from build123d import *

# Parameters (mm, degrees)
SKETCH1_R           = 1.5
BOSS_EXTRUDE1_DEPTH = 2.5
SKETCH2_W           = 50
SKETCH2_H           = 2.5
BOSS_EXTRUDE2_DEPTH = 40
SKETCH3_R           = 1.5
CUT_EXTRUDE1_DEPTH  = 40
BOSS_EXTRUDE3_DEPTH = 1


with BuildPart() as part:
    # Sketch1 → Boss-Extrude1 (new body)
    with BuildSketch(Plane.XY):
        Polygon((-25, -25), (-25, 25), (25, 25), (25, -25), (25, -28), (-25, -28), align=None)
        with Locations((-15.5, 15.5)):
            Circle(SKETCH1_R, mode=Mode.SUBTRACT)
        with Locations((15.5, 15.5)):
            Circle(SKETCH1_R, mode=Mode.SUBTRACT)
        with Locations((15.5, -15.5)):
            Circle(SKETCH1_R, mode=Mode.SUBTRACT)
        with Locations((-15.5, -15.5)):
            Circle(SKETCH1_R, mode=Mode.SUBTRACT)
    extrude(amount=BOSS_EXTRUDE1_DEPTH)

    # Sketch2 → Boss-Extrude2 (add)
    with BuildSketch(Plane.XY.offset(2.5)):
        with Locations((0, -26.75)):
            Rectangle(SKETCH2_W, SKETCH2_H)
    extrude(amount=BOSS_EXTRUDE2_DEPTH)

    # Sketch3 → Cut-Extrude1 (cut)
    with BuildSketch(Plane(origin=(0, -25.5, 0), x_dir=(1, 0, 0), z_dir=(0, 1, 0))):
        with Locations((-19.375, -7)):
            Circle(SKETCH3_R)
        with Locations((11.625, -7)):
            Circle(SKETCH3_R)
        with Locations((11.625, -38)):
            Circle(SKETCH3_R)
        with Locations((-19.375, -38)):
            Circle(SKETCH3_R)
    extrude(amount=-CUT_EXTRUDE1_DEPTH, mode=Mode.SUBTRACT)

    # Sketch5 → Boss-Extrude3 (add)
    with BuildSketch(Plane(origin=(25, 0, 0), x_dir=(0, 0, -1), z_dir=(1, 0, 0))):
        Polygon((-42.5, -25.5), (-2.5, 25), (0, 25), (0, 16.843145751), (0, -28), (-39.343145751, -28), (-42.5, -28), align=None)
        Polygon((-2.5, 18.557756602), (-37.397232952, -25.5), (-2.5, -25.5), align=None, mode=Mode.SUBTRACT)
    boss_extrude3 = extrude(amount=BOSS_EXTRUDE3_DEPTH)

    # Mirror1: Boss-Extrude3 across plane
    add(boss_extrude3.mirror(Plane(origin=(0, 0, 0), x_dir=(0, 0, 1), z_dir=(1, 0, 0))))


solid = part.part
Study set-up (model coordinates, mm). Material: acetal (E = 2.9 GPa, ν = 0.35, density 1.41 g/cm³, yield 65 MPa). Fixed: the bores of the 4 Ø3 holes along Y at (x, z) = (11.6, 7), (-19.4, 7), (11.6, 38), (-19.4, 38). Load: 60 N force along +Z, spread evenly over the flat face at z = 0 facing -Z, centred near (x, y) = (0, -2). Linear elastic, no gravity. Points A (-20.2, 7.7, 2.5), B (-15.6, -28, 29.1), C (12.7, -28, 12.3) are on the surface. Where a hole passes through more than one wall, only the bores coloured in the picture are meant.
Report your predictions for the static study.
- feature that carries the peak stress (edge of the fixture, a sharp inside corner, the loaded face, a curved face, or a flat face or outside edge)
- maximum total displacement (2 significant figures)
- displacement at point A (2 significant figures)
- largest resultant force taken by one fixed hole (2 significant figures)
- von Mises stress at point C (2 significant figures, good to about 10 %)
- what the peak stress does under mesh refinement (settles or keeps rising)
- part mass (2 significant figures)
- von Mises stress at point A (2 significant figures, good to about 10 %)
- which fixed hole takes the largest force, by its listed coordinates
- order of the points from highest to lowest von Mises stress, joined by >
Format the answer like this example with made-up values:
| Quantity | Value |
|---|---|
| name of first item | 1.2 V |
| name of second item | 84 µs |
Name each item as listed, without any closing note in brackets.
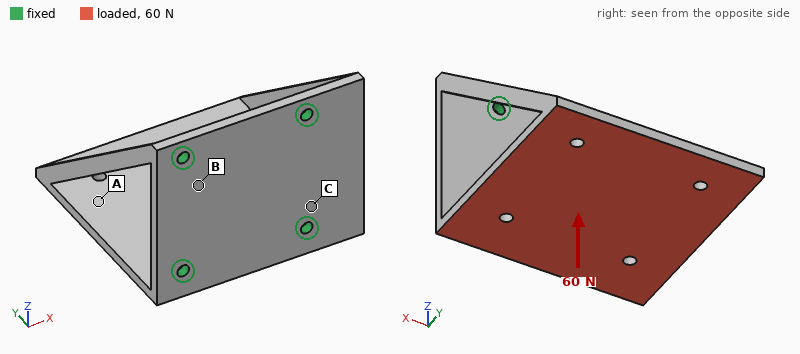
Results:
| Quantity | Value |
|---|---|
| feature that carries the peak stress | edge of the fixture |
| maximum total displacement | 0.86 mm |
| displacement at point A | 0.47 mm |
| largest resultant force taken by one fixed hole | 31 N |
| von Mises stress at point C | 2.0 MPa |
| what the peak stress does under mesh refinement | keeps rising |
| part mass | 18 g |
| von Mises stress at point A | 5.5 MPa |
| which fixed hole takes the largest force, by its listed coordinates | (11.6, 7) |
| order of the points from highest to lowest von Mises stress, joined by > | A > C > B |
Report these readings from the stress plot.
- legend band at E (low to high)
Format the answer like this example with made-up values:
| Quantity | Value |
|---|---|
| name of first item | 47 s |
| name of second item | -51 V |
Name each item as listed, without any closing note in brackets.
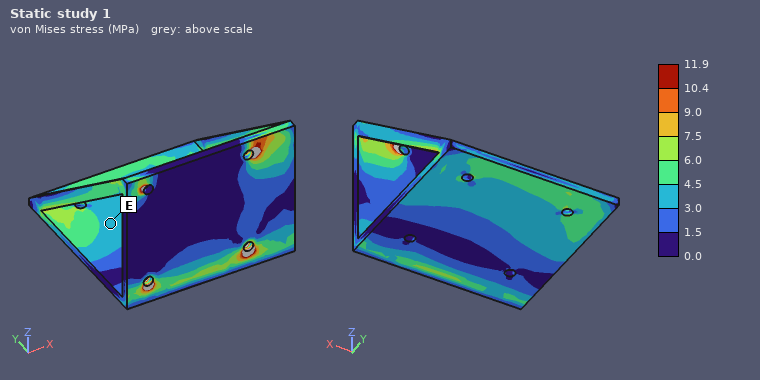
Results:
| Quantity | Value |
|---|---|
| legend band at E | 3.0 to 4.5 MPa |
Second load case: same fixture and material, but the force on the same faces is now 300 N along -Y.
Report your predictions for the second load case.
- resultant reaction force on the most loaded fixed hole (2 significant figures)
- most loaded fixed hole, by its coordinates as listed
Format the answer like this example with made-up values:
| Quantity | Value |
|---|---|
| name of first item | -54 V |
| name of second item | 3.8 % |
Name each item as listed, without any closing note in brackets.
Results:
| Quantity | Value |
|---|---|
| resultant reaction force on the most loaded fixed hole | 200 N |
| most loaded fixed hole, by its coordinates as listed | (11.6, 7) |
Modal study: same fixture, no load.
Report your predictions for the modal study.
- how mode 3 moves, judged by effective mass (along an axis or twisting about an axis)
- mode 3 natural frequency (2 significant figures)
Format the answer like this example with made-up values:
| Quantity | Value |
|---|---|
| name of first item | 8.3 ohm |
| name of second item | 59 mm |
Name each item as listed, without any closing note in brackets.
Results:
| Quantity | Value |
|---|---|
| how mode 3 moves, judged by effective mass | along Z |
| mode 3 natural frequency | 520 Hz |
